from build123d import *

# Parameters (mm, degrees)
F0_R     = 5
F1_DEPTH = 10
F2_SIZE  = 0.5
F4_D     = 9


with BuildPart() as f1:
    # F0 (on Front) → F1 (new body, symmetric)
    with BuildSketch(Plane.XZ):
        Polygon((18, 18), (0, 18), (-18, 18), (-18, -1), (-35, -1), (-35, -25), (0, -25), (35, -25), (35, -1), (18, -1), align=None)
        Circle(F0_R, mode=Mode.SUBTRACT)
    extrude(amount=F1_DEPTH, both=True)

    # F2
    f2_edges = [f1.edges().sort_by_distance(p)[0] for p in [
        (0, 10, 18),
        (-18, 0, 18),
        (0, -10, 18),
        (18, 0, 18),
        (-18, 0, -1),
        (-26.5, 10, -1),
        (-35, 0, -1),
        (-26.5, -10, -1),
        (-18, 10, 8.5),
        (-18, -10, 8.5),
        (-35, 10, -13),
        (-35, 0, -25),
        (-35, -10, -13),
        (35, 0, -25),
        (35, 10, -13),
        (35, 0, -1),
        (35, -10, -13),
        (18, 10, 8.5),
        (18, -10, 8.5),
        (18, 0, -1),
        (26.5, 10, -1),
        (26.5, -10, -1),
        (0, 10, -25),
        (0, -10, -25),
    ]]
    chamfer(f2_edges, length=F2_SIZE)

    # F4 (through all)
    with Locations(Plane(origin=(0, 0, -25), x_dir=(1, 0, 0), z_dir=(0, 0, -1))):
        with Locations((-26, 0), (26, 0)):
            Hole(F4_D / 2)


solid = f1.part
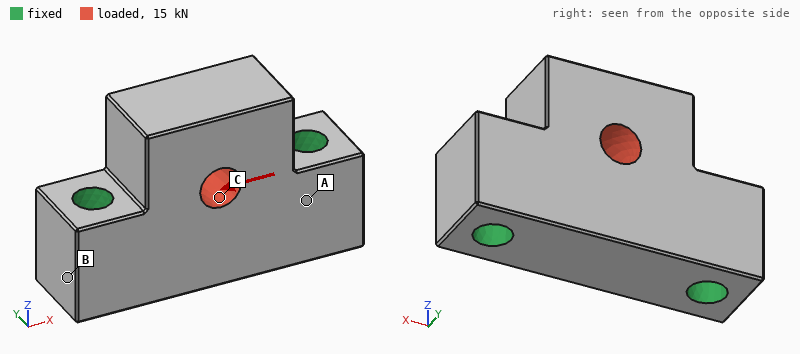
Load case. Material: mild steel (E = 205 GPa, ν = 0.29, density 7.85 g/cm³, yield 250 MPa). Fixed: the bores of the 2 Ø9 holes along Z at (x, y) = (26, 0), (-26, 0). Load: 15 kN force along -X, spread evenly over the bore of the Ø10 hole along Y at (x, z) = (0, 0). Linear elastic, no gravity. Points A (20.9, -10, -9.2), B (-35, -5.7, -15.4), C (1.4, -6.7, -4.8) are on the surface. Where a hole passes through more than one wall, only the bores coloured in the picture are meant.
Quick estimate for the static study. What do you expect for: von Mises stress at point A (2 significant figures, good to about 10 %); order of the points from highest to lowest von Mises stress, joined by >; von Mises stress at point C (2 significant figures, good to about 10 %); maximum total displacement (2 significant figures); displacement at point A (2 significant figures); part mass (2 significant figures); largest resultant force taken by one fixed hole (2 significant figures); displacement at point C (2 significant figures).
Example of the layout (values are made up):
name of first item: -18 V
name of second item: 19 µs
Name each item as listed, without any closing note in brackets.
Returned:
von Mises stress at point A: 14 MPa
order of the points from highest to lowest von Mises stress, joined by >: C > A > B
von Mises stress at point C: 43 MPa
maximum total displacement: 4.6 µm
displacement at point A: 0.75 µm
part mass: 330 g
largest resultant force taken by one fixed hole: 8.1 kN
displacement at point C: 2.3 µm
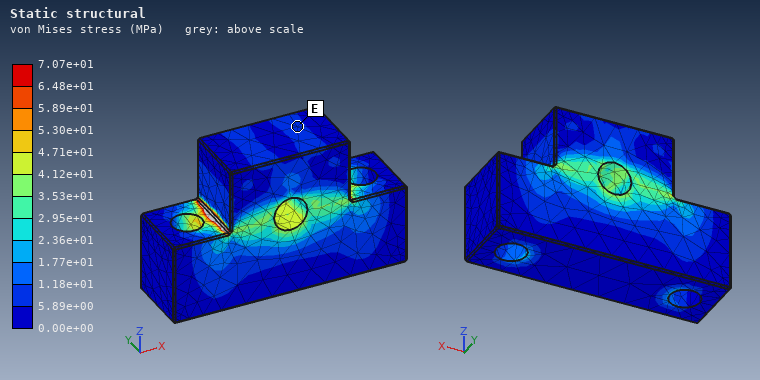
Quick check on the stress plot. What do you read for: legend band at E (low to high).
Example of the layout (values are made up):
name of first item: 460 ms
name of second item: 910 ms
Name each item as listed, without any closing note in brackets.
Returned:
legend band at E: 5.89e+00 to 1.18e+01 MPa
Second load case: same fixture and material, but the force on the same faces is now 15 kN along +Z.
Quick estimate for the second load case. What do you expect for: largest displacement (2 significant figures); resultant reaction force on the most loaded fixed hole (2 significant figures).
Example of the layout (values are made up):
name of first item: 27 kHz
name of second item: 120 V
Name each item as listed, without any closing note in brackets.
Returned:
largest displacement: 4.9 µm
resultant reaction force on the most loaded fixed hole: 7.8 kN
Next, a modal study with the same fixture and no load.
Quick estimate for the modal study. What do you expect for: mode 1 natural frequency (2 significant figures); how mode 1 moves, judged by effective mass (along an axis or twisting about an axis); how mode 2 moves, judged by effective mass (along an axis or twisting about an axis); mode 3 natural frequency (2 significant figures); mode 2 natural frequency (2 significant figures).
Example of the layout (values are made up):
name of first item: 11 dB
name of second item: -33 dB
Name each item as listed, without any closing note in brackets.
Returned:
mode 1 natural frequency: 11 kHz
how mode 1 moves, judged by effective mass: along Y
how mode 2 moves, judged by effective mass: along X
mode 3 natural frequency: 23 kHz
mode 2 natural frequency: 22 kHz
